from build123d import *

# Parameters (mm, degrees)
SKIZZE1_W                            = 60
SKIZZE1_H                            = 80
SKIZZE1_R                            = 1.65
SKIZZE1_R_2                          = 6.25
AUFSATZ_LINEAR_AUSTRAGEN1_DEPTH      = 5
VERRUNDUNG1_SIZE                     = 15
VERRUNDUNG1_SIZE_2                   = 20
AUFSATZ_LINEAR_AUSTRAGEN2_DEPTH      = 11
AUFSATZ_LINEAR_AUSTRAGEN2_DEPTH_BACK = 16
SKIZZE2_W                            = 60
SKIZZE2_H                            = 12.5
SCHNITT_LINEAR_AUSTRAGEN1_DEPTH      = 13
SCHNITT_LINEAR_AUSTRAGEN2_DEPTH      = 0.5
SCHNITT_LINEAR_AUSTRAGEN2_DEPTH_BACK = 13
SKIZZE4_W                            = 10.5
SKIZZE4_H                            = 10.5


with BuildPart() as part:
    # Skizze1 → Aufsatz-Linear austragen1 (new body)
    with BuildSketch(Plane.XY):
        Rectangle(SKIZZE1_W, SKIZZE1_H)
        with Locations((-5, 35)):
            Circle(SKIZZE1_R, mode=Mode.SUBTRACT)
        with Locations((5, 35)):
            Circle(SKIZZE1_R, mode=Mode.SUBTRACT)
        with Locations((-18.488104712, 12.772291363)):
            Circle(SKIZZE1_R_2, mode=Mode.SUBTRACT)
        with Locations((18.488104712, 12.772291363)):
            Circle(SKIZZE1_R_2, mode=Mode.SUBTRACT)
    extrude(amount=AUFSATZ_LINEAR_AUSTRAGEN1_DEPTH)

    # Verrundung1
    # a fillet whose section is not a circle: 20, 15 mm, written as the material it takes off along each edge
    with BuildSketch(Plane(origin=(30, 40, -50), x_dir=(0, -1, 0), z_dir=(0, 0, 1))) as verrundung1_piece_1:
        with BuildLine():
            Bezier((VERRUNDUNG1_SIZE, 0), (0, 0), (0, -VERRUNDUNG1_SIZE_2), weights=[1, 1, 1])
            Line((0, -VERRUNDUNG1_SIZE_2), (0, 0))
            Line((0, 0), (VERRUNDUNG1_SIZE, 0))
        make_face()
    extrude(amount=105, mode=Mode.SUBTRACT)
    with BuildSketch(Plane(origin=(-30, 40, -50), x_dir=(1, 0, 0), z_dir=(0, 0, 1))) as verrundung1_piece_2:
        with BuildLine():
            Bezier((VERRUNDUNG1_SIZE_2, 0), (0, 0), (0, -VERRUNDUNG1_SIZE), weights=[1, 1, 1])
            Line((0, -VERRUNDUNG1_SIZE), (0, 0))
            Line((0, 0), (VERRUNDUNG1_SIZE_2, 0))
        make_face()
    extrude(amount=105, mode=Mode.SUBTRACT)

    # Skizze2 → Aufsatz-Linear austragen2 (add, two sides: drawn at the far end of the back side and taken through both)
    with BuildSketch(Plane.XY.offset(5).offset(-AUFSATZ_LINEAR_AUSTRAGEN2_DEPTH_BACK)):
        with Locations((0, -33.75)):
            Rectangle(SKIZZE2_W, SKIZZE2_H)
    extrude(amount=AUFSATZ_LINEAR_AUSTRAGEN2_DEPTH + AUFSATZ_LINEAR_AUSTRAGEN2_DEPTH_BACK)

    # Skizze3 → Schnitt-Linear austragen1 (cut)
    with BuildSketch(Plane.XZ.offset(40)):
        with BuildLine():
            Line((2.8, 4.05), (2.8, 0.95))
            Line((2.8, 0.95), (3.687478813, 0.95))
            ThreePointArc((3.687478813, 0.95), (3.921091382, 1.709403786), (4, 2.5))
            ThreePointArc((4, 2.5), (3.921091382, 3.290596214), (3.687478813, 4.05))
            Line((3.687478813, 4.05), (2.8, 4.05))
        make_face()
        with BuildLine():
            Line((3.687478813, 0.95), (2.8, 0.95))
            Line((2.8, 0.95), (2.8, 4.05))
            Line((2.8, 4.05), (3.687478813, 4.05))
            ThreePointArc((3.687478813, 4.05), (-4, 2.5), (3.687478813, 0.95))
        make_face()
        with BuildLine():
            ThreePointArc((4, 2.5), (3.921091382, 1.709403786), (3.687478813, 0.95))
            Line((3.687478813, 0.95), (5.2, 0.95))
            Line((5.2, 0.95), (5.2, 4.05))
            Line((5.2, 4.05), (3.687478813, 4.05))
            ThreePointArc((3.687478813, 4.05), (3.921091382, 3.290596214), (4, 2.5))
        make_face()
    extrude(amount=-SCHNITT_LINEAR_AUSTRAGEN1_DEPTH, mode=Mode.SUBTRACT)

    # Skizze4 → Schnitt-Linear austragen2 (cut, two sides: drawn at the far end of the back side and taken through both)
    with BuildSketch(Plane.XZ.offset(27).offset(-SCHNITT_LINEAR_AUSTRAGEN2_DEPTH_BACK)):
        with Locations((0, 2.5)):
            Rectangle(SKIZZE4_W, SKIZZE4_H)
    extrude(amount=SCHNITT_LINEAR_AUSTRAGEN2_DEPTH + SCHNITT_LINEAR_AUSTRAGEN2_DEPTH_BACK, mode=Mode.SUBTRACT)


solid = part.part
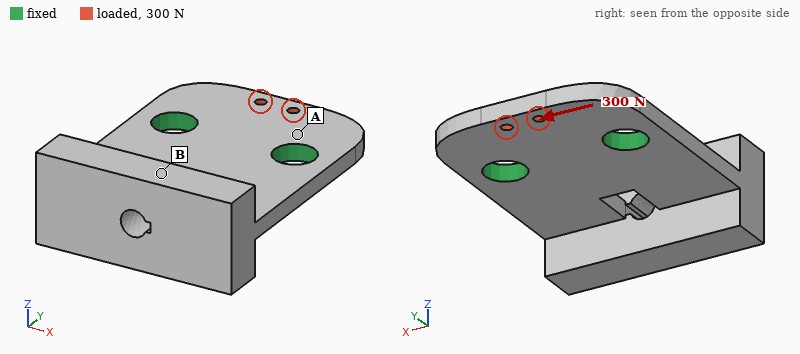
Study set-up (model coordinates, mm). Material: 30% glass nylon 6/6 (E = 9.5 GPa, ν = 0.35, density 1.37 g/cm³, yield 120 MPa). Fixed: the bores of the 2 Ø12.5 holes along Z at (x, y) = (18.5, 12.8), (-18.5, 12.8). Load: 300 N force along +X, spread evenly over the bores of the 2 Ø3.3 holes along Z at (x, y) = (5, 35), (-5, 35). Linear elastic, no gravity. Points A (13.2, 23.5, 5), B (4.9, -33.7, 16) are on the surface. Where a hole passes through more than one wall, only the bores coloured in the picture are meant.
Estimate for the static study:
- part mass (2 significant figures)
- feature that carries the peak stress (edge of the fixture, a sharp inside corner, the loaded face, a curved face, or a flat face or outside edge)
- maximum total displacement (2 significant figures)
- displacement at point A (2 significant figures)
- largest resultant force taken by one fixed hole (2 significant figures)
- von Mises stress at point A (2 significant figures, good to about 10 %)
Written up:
51 g
the loaded face
9.3 µm
2.4 µm
200 N
2.4 MPa
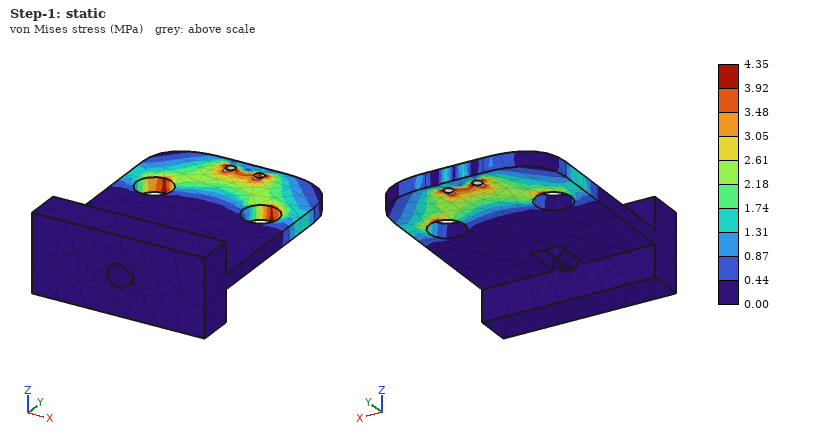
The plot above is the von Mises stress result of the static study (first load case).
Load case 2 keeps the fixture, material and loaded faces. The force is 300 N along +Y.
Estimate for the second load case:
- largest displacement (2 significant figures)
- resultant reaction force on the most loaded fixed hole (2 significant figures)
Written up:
6.6 µm
160 N
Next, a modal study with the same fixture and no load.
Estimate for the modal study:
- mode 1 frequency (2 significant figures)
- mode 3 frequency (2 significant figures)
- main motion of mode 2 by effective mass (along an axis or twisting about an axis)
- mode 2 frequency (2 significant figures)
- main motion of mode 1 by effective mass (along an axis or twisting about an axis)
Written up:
440 Hz
2800 Hz
twisting about Y
1200 Hz
along Z
